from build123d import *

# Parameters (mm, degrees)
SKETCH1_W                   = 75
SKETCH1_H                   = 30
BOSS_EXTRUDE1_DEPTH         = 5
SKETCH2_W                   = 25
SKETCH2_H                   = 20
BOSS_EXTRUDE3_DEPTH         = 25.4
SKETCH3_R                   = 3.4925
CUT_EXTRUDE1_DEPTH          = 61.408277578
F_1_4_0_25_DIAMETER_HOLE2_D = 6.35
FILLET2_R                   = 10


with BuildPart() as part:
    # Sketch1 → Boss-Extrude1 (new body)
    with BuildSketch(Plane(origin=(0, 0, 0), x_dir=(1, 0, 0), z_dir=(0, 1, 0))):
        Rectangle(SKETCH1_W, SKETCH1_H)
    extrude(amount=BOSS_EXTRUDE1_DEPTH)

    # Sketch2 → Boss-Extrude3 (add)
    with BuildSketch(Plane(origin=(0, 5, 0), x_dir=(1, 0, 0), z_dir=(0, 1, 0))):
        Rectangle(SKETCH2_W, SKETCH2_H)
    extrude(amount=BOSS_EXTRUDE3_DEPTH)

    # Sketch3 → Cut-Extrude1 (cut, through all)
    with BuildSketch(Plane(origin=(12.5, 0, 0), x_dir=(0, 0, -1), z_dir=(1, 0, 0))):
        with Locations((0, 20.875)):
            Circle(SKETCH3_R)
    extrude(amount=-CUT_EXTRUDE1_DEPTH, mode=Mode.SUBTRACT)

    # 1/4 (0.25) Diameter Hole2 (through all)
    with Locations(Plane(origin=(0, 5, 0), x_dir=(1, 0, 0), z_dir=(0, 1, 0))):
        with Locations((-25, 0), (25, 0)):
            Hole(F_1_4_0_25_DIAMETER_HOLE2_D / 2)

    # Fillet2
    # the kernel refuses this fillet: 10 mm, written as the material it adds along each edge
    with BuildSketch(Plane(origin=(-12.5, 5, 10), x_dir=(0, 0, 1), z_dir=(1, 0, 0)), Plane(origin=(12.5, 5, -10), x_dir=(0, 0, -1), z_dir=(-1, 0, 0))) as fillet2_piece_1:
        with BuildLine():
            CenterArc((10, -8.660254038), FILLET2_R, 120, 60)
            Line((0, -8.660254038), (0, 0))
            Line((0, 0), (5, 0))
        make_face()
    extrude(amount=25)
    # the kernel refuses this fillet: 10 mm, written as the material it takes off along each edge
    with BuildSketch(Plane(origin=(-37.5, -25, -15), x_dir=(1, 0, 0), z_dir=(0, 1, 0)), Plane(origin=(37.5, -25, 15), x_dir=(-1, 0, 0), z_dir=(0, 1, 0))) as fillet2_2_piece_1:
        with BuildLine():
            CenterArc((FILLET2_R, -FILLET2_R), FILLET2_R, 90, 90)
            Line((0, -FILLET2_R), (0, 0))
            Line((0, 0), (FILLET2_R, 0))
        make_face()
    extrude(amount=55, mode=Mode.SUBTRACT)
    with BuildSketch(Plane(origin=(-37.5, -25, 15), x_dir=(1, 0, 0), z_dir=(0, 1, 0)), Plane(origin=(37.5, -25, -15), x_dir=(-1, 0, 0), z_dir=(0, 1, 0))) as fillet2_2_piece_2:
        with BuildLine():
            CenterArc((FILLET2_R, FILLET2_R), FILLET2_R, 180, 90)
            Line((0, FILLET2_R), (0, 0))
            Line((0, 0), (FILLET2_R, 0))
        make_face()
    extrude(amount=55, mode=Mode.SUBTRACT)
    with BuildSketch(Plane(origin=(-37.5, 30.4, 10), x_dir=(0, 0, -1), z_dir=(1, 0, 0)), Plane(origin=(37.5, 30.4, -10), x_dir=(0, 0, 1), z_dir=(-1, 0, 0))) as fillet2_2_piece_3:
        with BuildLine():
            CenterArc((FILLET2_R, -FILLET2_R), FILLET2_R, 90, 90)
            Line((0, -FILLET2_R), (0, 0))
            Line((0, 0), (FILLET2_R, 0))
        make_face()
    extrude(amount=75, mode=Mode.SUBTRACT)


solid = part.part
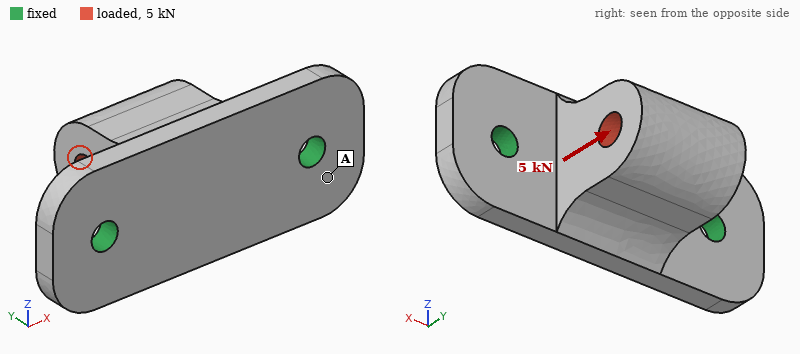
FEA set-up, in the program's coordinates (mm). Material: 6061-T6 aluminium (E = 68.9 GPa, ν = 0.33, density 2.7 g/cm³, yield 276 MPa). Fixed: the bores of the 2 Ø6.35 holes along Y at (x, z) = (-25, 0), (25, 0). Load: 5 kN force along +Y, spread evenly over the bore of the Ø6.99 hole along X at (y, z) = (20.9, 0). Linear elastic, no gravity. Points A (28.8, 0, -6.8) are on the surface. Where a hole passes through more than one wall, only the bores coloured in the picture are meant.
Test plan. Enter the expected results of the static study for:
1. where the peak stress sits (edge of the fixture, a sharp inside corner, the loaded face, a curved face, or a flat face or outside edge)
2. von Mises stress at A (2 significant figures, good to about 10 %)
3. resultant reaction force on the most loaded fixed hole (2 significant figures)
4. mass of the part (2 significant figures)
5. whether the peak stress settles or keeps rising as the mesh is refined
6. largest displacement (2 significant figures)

edge of the fixture
30 MPa
2.7 kN
59 g
keeps rising
51 µm
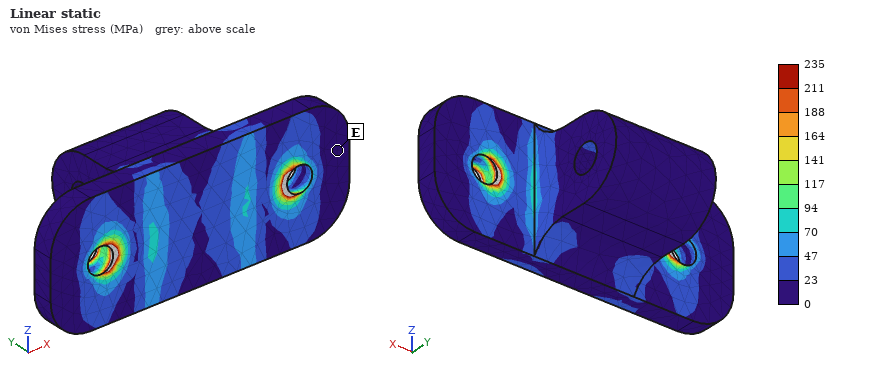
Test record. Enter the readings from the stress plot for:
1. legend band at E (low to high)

0 to 23 MPa
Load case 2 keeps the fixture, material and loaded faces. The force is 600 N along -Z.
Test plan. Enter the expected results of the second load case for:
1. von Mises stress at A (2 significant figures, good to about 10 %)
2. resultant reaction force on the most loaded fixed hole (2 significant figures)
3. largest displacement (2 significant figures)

17 MPa
300 N
53 µm
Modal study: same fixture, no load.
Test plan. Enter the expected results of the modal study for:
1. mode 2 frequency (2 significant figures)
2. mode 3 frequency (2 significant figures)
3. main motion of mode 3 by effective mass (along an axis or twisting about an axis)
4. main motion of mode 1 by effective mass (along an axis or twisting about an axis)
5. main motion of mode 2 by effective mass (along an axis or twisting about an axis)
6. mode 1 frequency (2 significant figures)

7800 Hz
9200 Hz
along X
along Z
along Y
4000 Hz
